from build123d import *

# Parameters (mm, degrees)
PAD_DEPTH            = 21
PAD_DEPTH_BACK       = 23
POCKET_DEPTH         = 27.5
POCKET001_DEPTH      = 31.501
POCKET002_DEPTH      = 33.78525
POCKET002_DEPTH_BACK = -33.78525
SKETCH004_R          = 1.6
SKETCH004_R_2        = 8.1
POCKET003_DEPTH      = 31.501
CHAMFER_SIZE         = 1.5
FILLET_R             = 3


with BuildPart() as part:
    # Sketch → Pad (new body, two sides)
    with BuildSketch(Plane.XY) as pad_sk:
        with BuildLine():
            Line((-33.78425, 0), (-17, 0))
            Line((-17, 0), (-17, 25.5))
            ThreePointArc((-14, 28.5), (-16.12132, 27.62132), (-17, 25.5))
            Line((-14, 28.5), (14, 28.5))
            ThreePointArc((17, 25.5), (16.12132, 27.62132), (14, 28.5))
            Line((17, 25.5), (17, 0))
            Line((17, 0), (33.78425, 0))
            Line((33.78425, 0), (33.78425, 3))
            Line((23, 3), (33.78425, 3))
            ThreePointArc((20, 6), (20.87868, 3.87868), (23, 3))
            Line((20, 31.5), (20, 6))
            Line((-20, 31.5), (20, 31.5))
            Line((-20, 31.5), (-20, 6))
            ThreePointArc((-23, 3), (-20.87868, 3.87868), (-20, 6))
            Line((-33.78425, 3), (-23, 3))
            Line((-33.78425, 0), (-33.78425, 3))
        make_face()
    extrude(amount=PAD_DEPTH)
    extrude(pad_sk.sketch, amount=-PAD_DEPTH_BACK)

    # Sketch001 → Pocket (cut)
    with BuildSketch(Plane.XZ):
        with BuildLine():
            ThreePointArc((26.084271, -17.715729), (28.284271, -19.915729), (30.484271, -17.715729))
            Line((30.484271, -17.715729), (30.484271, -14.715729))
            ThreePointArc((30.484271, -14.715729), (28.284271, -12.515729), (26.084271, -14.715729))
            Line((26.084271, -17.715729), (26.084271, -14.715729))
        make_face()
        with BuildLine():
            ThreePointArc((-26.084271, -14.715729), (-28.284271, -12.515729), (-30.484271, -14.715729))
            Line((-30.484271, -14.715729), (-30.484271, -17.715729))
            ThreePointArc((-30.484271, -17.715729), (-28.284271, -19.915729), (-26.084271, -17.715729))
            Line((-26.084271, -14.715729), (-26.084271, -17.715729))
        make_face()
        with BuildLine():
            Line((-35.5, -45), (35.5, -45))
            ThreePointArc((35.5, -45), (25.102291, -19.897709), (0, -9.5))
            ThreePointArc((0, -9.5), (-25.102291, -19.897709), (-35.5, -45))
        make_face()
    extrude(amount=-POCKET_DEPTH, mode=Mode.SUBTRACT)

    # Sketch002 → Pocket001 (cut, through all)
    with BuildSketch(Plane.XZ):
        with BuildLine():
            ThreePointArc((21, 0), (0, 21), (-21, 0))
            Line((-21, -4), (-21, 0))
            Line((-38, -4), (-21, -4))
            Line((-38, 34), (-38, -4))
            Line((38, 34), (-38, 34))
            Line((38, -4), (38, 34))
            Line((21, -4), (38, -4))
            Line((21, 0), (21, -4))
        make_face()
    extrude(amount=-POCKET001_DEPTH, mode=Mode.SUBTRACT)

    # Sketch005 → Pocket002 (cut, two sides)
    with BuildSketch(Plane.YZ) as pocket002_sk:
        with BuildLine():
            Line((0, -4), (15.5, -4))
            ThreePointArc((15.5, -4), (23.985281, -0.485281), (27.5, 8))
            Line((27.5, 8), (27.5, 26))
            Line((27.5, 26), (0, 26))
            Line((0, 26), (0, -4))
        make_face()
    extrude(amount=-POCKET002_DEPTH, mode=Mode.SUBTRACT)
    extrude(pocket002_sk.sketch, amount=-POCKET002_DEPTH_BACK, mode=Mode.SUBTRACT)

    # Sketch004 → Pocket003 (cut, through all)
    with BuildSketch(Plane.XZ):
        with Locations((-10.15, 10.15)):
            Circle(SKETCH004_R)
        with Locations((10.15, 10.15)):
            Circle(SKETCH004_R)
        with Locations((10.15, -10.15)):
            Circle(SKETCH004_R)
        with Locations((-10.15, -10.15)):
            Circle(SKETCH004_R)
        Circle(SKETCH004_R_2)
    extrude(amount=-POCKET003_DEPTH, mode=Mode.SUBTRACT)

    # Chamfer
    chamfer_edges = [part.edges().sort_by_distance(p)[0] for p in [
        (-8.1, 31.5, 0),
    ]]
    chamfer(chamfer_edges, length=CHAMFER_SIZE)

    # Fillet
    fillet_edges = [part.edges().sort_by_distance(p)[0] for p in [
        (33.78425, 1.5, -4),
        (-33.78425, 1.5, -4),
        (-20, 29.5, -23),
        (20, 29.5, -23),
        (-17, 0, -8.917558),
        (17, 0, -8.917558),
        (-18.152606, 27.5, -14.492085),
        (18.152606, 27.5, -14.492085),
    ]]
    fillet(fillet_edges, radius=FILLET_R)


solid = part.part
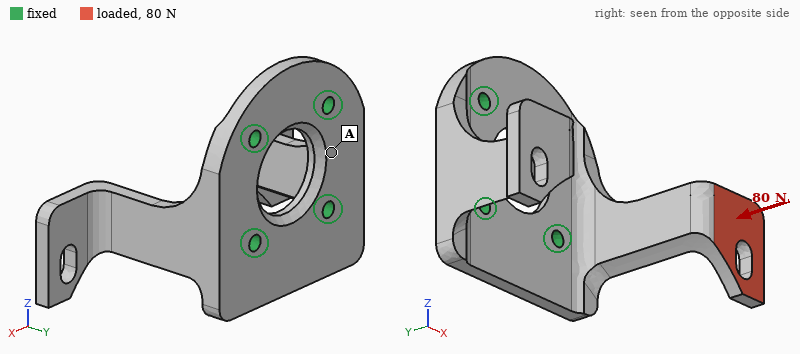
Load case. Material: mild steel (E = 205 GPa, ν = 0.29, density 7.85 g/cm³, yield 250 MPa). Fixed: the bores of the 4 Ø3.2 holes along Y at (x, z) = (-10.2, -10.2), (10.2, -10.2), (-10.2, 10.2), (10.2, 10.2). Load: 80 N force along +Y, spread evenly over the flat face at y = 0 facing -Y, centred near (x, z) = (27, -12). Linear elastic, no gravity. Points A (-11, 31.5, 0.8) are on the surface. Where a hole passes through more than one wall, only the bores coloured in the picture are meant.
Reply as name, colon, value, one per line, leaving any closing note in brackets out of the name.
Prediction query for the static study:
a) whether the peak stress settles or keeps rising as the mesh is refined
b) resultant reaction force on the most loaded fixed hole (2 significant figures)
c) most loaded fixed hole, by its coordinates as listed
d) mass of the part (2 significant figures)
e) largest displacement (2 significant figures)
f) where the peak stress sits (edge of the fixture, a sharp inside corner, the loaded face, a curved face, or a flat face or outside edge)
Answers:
whether the peak stress settles or keeps rising as the mesh is refined: keeps rising
resultant reaction force on the most loaded fixed hole: 91 N
most loaded fixed hole, by its coordinates as listed: (10.2, -10.2)
mass of the part: 59 g
largest displacement: 99 µm
where the peak stress sits: edge of the fixture
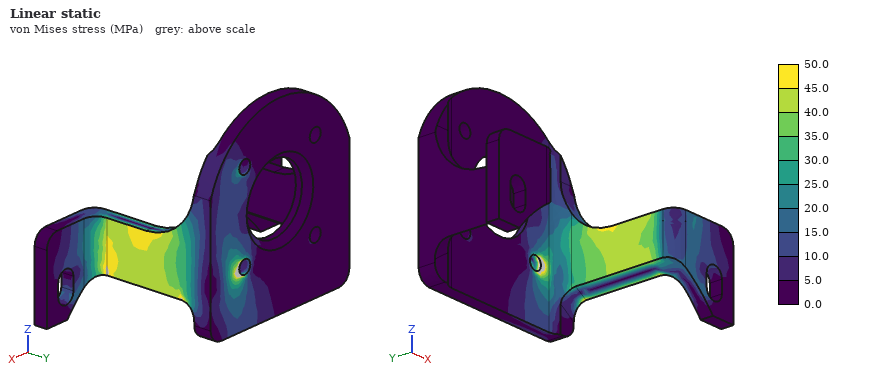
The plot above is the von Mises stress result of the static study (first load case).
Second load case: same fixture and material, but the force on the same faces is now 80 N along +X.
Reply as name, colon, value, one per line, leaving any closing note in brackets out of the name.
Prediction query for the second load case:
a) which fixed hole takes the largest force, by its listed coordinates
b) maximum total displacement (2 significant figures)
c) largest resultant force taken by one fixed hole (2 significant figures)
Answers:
which fixed hole takes the largest force, by its listed coordinates: (10.2, -10.2)
maximum total displacement: 0.19 mm
largest resultant force taken by one fixed hole: 85 N
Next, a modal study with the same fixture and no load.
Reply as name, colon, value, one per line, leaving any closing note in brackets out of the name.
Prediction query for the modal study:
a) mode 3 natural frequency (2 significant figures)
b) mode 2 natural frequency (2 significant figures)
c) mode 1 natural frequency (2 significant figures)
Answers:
mode 3 natural frequency: 3200 Hz
mode 2 natural frequency: 1400 Hz
mode 1 natural frequency: 1400 Hz
